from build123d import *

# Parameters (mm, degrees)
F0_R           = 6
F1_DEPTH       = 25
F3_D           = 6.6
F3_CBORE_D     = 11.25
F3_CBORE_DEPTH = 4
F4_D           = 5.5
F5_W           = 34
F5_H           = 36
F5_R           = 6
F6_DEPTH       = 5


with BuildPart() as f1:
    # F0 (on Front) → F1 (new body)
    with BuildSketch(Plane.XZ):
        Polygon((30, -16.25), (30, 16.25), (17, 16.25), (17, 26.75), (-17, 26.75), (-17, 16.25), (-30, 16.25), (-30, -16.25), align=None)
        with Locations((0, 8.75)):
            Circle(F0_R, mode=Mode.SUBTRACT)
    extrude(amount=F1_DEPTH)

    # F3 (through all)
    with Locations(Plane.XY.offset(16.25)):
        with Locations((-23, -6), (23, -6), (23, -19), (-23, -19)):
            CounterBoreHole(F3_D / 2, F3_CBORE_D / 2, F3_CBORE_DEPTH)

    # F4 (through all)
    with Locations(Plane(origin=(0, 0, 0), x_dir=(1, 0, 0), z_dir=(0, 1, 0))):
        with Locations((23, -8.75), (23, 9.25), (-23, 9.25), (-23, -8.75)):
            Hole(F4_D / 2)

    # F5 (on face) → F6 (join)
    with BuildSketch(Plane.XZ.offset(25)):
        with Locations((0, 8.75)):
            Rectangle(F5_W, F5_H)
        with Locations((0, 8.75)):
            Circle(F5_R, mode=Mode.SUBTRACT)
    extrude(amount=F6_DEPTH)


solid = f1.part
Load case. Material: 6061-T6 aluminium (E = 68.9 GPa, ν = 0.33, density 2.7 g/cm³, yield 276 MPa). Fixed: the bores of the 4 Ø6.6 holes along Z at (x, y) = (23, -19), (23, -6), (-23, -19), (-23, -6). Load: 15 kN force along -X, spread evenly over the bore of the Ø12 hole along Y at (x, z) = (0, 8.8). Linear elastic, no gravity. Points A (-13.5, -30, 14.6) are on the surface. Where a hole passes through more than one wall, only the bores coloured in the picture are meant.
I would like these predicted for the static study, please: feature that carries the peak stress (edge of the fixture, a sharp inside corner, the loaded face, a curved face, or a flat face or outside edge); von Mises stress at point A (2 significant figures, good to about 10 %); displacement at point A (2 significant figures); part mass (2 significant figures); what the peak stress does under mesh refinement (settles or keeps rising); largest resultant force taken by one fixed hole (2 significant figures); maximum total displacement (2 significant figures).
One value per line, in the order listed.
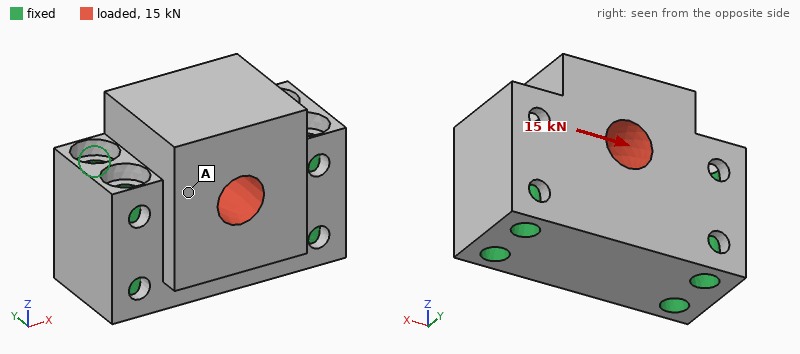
edge of the fixture
7.1 MPa
5.1 µm
140 g
keeps rising
4.3 kN
6.6 µm
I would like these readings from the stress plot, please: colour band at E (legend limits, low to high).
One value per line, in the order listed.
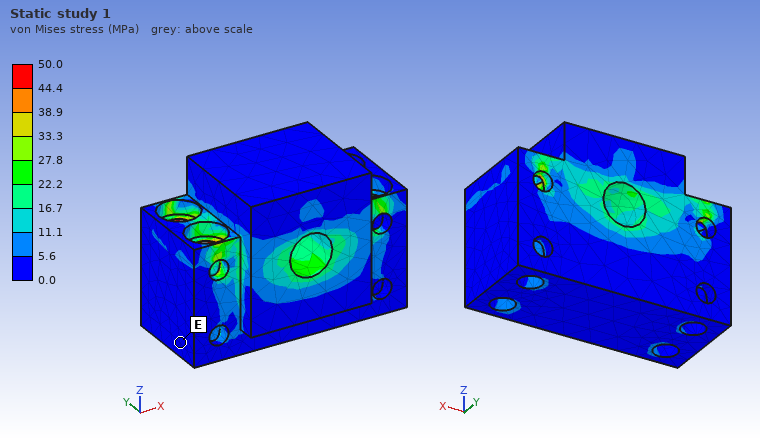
0.0 to 5.6 MPa
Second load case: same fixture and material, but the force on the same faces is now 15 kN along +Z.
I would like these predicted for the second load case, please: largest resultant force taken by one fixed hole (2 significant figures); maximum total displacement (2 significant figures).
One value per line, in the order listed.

4.5 kN
10 µm
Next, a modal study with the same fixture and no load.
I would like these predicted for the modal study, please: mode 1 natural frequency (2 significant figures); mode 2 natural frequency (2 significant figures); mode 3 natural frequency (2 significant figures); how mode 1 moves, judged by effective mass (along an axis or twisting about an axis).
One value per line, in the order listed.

17 kHz
28 kHz
29 kHz
along Y
